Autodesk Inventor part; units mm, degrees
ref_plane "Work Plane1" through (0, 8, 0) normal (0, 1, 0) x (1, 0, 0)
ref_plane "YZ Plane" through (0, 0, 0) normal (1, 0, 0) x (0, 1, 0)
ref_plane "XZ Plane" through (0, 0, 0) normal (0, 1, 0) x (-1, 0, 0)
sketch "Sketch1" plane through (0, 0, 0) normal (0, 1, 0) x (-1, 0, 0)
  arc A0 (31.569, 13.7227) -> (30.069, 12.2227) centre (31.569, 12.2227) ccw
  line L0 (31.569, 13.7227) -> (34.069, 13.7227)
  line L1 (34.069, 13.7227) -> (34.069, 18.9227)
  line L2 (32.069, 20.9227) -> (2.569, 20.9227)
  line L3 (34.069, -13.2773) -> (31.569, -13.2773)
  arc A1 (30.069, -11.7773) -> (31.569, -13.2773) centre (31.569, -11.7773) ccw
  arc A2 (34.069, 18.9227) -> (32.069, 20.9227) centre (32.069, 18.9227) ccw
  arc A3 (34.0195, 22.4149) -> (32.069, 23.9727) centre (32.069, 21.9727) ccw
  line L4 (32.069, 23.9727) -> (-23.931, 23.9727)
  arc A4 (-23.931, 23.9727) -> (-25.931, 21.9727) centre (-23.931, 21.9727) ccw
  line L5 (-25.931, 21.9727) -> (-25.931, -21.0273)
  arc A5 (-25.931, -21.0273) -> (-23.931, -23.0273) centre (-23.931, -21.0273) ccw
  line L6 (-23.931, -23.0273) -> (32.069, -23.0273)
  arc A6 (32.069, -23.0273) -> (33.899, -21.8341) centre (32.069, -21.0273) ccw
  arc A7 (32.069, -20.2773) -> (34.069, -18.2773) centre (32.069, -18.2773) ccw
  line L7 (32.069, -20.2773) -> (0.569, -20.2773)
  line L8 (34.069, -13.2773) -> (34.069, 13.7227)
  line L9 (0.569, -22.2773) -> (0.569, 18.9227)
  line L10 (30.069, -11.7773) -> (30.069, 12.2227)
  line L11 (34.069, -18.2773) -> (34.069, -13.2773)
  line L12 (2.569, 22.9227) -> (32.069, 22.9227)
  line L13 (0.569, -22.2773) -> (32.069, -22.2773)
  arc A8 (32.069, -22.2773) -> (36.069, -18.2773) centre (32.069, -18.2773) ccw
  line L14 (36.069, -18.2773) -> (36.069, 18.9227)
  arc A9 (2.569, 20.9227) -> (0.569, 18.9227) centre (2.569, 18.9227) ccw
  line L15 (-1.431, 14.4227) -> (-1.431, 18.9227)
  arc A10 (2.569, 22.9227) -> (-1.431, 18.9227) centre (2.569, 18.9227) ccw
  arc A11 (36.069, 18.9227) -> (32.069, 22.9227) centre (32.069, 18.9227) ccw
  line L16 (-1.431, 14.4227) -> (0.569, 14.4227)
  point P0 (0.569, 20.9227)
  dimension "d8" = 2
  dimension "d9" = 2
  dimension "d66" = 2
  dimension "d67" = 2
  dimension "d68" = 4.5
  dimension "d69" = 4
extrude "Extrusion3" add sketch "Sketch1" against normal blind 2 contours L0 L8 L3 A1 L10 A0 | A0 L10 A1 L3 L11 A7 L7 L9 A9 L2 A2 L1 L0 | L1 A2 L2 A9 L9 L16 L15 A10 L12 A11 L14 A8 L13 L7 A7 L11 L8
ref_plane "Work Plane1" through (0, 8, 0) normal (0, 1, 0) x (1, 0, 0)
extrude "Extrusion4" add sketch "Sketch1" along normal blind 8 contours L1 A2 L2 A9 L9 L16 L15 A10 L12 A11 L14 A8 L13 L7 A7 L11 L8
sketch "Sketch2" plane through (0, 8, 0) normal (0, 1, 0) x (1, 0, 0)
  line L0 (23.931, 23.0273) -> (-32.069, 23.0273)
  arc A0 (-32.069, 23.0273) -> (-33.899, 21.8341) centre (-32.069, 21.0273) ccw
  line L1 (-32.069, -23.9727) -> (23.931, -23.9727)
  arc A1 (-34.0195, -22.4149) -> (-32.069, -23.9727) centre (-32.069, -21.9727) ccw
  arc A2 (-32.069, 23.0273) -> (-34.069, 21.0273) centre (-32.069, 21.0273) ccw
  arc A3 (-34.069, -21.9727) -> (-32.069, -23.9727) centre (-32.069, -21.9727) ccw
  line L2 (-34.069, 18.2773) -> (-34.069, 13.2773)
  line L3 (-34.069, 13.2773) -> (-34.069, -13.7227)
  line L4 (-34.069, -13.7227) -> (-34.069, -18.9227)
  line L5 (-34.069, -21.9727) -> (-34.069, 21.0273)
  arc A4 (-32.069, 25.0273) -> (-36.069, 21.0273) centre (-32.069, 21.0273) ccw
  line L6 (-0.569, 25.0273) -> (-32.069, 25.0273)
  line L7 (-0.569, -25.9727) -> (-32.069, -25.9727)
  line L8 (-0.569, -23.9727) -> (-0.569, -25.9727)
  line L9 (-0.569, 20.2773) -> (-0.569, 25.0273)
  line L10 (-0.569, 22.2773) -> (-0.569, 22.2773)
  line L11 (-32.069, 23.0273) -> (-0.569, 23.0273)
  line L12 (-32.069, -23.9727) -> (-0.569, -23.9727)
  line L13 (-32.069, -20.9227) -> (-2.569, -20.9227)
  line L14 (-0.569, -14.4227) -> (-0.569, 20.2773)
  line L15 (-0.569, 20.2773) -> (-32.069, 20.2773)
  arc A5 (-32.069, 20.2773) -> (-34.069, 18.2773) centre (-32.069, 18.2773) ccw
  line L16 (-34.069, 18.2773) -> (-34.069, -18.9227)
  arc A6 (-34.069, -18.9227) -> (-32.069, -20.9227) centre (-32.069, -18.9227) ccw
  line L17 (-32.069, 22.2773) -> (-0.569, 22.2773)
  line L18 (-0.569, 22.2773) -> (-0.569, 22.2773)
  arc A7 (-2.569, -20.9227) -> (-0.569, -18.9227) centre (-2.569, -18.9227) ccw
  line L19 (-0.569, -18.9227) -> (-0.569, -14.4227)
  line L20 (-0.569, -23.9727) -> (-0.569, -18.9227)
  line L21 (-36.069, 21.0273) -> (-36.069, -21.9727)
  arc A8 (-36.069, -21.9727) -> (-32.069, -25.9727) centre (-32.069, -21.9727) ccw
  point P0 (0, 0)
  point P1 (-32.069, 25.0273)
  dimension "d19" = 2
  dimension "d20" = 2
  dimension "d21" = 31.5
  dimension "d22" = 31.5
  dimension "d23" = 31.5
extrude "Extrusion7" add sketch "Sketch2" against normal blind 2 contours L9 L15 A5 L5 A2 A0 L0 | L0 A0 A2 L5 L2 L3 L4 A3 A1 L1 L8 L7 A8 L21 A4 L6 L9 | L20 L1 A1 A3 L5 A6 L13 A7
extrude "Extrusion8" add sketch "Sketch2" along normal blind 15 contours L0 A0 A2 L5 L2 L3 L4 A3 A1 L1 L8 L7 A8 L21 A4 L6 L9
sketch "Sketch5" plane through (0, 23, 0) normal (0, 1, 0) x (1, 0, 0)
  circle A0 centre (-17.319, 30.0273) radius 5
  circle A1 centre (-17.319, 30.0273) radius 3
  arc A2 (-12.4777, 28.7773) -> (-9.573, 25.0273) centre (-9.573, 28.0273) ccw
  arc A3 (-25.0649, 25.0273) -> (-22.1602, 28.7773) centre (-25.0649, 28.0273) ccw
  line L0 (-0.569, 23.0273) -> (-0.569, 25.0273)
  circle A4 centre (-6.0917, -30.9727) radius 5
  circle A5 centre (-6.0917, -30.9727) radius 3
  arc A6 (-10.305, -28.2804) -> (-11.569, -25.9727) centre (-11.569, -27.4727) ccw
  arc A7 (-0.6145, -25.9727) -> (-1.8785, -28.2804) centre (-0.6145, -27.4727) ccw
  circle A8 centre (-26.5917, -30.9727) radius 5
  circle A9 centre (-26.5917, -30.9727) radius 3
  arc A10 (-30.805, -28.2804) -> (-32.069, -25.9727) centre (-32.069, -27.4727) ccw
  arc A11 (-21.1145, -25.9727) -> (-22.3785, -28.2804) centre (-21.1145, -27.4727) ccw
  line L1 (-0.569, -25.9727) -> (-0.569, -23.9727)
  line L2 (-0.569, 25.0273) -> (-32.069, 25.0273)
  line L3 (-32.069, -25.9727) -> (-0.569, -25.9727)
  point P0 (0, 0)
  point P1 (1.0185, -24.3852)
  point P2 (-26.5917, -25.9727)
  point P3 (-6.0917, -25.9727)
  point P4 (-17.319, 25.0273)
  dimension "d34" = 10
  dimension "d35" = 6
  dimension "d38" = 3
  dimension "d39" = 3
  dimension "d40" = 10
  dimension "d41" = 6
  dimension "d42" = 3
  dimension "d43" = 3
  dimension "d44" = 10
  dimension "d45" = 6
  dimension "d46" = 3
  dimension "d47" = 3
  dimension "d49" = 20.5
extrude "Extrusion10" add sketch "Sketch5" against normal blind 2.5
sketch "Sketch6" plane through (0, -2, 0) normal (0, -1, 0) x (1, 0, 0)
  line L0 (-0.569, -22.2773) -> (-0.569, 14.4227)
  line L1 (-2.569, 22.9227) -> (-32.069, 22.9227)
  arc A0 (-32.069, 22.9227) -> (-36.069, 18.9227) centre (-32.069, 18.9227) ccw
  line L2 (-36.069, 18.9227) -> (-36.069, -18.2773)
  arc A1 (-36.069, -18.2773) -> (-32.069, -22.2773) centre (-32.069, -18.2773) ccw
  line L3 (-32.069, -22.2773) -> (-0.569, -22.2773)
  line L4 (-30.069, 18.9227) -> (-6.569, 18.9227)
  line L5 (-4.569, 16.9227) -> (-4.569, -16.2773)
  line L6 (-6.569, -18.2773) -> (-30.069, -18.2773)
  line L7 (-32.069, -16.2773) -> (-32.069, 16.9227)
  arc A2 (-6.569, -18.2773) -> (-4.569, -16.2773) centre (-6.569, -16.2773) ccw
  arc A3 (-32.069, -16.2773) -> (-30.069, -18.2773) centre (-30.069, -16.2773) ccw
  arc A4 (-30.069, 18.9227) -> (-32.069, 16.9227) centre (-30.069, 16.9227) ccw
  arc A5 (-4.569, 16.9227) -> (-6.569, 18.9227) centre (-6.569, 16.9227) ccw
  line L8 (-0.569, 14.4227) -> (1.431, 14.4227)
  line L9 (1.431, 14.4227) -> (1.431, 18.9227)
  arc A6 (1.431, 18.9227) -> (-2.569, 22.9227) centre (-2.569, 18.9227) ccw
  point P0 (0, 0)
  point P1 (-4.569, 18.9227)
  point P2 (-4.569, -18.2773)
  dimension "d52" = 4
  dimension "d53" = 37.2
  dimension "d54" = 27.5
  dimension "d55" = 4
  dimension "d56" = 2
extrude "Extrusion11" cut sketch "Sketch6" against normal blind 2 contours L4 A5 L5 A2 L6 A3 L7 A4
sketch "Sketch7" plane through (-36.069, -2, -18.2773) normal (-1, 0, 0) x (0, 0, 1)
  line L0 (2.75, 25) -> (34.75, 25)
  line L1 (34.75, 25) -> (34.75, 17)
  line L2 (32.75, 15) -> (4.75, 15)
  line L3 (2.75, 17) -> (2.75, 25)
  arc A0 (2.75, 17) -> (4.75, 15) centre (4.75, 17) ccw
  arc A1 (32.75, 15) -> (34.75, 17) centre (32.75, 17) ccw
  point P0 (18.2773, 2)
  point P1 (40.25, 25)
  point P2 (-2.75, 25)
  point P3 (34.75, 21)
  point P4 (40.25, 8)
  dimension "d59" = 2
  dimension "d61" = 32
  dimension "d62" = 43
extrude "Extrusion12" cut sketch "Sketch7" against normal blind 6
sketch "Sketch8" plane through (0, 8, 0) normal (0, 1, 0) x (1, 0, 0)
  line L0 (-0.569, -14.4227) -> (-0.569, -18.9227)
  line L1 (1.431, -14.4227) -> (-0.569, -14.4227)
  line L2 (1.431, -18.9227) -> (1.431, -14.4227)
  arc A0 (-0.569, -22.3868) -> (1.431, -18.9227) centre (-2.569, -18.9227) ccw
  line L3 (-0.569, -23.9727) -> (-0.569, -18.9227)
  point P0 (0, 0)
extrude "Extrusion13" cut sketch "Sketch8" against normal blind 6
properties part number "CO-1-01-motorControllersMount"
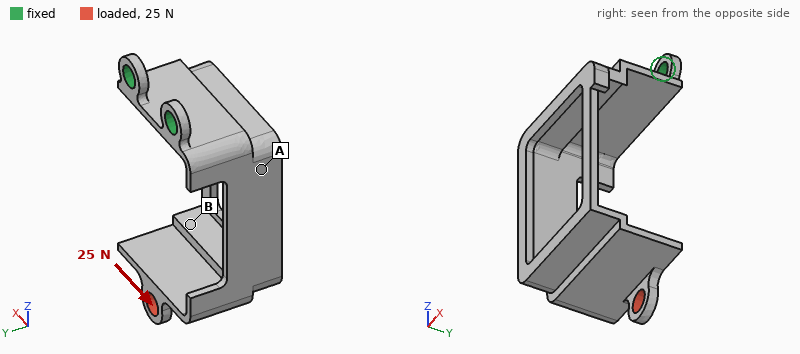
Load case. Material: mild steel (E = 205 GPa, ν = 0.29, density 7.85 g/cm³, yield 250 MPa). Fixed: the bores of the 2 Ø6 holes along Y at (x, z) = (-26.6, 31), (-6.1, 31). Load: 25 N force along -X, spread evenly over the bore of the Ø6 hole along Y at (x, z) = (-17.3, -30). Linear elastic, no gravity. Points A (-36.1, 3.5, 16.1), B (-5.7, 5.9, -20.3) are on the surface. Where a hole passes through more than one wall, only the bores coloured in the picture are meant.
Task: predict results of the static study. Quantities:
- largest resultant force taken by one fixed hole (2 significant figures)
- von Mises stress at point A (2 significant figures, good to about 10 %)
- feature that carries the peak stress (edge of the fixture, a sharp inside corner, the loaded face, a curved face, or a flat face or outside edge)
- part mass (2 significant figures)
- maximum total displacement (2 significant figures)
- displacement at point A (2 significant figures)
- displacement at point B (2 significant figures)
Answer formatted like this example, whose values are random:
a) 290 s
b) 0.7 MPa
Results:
a) 51 N
b) 19 MPa
c) a curved face
d) 52 g
e) 0.23 mm
f) 0.038 mm
g) 0.14 mm
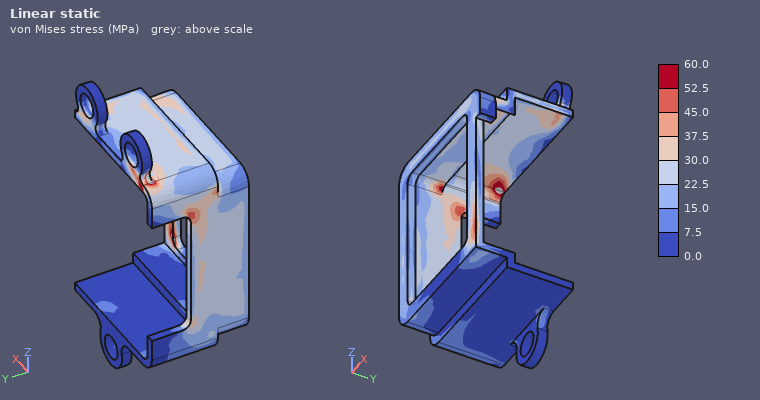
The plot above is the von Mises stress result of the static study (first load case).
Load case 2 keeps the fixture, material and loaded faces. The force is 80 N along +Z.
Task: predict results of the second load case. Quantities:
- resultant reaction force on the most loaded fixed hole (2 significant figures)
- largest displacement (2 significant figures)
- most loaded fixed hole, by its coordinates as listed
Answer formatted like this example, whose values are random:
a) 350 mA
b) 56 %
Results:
a) 48 N
b) 0.24 mm
c) (-6.1, 31)
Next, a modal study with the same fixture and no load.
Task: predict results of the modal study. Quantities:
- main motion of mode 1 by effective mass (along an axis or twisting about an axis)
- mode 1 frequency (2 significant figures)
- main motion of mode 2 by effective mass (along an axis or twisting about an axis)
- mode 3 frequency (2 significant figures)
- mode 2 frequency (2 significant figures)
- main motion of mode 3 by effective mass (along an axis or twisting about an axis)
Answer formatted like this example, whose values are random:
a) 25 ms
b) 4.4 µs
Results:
a) along Y
b) 360 Hz
c) along X
d) 1200 Hz
e) 480 Hz
f) along Z
